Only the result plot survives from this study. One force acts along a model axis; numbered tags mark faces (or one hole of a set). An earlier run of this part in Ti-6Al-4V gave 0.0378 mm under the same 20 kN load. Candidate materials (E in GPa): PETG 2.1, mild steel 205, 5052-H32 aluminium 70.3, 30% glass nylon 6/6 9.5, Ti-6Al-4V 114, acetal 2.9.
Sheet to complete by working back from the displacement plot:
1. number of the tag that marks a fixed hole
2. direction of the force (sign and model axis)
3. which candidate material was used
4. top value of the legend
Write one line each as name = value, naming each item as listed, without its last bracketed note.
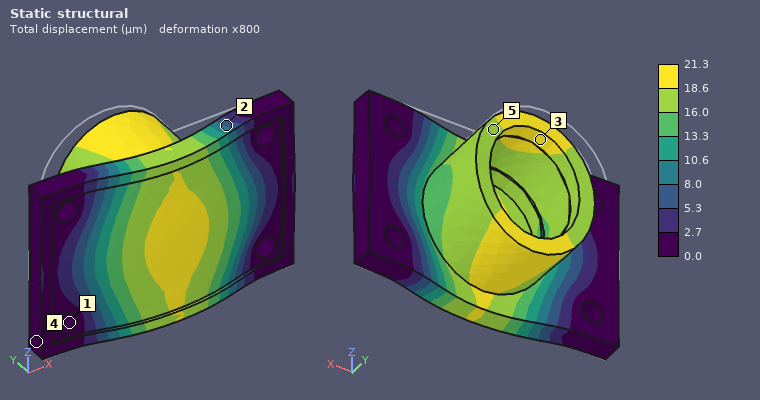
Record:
number of the tag that marks a fixed hole = 1
direction of the force = -Y
which candidate material was used = mild steel
top value of the legend = 21.3 µm
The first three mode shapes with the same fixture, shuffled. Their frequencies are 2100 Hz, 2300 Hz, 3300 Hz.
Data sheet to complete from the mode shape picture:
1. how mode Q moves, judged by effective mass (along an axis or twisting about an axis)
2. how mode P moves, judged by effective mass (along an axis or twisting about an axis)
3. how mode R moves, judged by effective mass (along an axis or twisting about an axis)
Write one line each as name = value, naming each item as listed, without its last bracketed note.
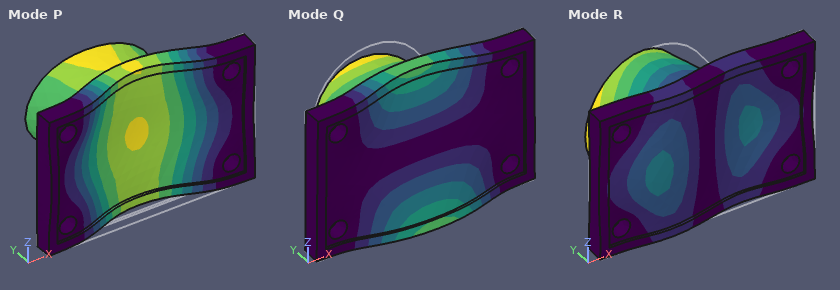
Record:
how mode Q moves, judged by effective mass = along Z
how mode P moves, judged by effective mass = along Y
how mode R moves, judged by effective mass = along X
